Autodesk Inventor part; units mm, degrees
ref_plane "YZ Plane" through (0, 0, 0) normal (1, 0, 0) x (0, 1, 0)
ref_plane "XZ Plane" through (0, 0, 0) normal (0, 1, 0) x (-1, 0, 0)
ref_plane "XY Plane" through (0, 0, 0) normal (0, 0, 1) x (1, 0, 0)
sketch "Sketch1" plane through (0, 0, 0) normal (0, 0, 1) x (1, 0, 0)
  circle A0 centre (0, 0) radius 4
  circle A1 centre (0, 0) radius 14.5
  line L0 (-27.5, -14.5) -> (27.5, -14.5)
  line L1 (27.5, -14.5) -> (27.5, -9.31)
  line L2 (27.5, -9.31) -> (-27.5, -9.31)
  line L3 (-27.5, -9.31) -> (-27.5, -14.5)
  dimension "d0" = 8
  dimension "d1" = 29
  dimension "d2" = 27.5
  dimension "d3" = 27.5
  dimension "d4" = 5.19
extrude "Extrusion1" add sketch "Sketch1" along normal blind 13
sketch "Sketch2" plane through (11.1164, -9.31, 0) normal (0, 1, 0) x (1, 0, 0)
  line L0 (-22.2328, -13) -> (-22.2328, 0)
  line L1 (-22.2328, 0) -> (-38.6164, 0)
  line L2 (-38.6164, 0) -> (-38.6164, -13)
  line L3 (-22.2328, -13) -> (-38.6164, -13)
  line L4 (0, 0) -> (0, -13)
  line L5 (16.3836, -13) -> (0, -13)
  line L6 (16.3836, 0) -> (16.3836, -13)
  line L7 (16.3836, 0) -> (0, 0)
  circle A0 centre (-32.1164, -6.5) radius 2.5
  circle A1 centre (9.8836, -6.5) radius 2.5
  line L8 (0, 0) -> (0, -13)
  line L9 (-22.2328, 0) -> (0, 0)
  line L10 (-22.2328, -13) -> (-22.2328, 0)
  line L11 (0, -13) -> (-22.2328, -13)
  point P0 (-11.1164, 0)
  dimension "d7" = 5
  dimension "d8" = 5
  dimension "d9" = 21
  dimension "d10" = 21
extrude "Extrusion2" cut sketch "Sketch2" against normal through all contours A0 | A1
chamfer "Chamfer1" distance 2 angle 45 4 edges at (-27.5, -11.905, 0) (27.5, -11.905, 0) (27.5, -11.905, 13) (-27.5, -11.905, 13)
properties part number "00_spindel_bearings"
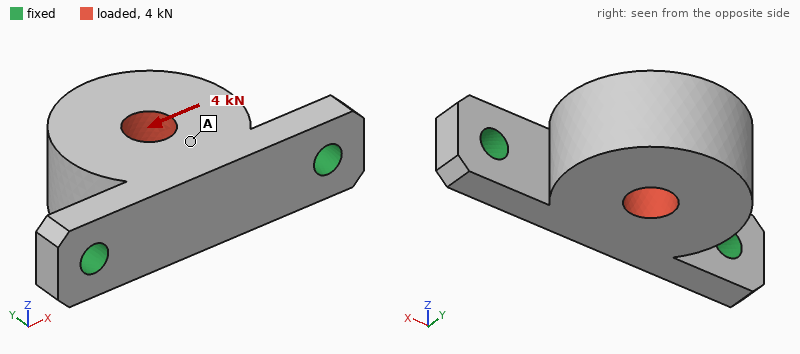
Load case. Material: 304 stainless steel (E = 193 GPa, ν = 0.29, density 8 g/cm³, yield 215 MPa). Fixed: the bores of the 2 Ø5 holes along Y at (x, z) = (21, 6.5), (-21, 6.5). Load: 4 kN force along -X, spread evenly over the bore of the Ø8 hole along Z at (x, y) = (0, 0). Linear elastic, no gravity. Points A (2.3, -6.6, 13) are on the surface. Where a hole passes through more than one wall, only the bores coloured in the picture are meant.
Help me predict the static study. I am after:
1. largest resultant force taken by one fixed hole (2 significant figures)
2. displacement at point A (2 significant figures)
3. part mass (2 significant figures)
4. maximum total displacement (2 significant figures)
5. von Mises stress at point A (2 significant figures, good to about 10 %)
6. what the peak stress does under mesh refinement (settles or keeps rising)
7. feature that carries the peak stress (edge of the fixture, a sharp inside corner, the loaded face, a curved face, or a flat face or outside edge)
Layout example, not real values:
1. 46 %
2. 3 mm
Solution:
1. 2.5 kN
2. 5.4 µm
3. 83 g
4. 21 µm
5. 29 MPa
6. keeps rising
7. edge of the fixture
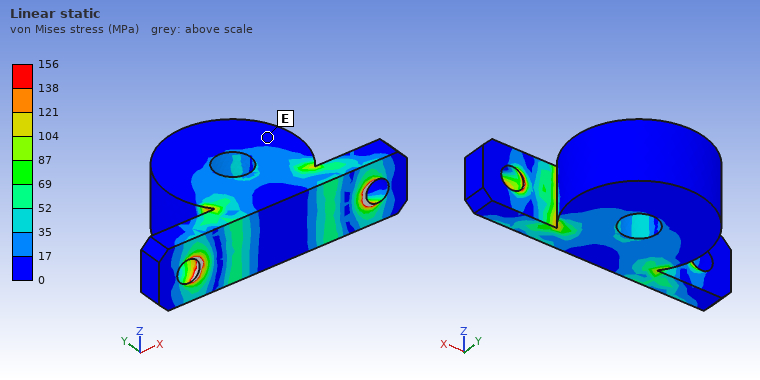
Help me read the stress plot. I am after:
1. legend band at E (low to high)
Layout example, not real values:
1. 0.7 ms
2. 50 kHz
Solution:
1. 0 to 17 MPa
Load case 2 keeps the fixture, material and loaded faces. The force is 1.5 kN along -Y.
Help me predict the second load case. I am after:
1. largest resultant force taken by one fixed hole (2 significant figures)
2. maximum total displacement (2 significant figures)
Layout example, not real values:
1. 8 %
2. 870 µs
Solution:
1. 810 N
2. 5.4 µm
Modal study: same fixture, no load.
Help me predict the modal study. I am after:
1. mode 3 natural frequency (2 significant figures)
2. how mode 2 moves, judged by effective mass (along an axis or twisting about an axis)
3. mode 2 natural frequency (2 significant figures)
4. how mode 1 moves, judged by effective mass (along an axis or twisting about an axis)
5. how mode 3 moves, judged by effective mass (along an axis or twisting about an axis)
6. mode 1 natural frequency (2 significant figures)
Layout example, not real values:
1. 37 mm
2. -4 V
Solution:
1. 10 kHz
2. along X
3. 9500 Hz
4. along Z
5. along Y
6. 3700 Hz
